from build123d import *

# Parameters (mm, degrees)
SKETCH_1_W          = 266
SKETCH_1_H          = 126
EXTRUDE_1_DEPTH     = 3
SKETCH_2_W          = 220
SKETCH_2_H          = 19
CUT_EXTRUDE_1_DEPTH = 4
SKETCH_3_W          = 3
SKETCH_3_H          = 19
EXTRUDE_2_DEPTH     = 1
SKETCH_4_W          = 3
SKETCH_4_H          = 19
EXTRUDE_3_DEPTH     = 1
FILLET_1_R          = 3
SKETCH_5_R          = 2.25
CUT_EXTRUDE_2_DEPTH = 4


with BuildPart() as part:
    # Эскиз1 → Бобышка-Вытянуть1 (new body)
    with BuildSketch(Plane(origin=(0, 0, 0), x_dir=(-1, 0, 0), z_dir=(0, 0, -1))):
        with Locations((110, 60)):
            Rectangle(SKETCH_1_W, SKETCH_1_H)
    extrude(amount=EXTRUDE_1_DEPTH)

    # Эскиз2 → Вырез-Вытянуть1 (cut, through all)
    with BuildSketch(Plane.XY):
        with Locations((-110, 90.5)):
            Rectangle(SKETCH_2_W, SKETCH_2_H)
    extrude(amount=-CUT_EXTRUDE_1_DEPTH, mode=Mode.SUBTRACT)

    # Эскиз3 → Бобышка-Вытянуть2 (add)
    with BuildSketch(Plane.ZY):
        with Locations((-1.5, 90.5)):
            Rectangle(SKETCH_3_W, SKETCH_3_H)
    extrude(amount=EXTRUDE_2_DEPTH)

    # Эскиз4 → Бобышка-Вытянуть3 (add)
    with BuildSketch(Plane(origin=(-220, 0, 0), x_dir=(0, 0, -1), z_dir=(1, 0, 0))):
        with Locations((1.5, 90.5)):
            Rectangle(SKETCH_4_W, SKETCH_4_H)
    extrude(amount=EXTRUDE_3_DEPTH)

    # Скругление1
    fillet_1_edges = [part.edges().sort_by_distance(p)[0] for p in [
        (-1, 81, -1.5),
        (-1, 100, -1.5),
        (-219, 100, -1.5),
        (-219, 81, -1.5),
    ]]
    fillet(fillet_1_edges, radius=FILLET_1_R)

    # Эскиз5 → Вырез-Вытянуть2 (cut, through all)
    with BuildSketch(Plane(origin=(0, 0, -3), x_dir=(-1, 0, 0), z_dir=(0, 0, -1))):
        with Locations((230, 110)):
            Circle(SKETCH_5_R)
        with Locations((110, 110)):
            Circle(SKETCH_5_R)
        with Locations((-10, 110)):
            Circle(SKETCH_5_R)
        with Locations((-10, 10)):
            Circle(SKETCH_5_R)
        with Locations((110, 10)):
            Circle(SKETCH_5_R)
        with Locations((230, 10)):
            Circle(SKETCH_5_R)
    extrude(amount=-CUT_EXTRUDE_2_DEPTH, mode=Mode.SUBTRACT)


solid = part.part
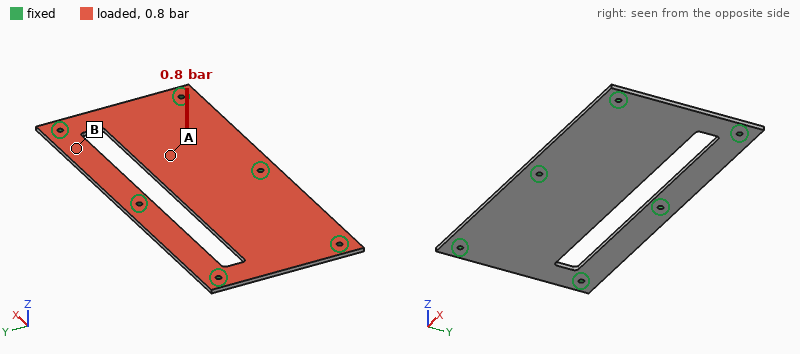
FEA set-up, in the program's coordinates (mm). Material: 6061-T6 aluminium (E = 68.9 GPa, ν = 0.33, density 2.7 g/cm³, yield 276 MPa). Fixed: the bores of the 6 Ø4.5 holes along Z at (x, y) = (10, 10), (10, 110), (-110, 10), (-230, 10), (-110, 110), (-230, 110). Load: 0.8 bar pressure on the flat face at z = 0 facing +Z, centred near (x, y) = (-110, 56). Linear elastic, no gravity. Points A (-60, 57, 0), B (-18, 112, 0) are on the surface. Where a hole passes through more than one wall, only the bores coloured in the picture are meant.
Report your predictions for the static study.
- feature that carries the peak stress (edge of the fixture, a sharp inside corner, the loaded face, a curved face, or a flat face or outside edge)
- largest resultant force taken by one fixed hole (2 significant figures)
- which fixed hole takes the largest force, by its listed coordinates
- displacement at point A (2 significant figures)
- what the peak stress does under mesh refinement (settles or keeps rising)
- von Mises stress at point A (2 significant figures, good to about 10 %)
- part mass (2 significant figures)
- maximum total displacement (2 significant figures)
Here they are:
edge of the fixture
810 N
(-110, 10)
1.1 mm
keeps rising
49 MPa
240 g
1.9 mm
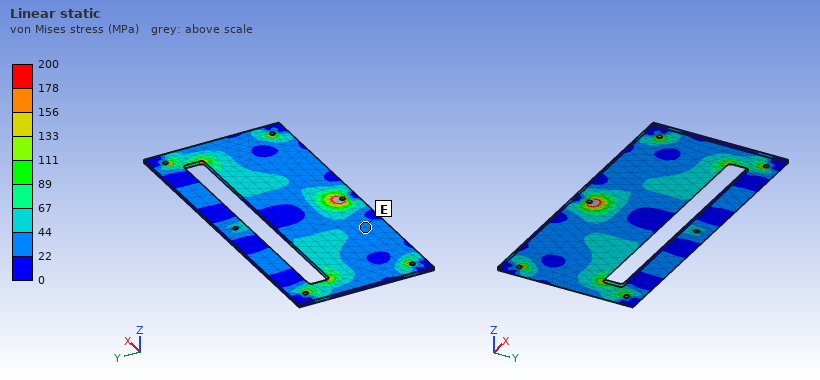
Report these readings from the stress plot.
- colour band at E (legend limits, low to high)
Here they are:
22 to 44 MPa
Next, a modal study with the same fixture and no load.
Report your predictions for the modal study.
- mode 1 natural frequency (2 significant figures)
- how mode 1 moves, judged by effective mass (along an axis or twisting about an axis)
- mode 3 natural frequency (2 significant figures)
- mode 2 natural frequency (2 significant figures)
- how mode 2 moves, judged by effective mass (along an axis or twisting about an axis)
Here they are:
490 Hz
along Z
1100 Hz
710 Hz
twisting about Y
